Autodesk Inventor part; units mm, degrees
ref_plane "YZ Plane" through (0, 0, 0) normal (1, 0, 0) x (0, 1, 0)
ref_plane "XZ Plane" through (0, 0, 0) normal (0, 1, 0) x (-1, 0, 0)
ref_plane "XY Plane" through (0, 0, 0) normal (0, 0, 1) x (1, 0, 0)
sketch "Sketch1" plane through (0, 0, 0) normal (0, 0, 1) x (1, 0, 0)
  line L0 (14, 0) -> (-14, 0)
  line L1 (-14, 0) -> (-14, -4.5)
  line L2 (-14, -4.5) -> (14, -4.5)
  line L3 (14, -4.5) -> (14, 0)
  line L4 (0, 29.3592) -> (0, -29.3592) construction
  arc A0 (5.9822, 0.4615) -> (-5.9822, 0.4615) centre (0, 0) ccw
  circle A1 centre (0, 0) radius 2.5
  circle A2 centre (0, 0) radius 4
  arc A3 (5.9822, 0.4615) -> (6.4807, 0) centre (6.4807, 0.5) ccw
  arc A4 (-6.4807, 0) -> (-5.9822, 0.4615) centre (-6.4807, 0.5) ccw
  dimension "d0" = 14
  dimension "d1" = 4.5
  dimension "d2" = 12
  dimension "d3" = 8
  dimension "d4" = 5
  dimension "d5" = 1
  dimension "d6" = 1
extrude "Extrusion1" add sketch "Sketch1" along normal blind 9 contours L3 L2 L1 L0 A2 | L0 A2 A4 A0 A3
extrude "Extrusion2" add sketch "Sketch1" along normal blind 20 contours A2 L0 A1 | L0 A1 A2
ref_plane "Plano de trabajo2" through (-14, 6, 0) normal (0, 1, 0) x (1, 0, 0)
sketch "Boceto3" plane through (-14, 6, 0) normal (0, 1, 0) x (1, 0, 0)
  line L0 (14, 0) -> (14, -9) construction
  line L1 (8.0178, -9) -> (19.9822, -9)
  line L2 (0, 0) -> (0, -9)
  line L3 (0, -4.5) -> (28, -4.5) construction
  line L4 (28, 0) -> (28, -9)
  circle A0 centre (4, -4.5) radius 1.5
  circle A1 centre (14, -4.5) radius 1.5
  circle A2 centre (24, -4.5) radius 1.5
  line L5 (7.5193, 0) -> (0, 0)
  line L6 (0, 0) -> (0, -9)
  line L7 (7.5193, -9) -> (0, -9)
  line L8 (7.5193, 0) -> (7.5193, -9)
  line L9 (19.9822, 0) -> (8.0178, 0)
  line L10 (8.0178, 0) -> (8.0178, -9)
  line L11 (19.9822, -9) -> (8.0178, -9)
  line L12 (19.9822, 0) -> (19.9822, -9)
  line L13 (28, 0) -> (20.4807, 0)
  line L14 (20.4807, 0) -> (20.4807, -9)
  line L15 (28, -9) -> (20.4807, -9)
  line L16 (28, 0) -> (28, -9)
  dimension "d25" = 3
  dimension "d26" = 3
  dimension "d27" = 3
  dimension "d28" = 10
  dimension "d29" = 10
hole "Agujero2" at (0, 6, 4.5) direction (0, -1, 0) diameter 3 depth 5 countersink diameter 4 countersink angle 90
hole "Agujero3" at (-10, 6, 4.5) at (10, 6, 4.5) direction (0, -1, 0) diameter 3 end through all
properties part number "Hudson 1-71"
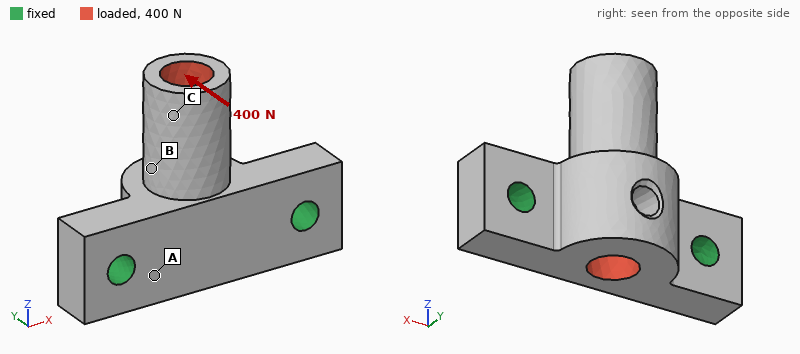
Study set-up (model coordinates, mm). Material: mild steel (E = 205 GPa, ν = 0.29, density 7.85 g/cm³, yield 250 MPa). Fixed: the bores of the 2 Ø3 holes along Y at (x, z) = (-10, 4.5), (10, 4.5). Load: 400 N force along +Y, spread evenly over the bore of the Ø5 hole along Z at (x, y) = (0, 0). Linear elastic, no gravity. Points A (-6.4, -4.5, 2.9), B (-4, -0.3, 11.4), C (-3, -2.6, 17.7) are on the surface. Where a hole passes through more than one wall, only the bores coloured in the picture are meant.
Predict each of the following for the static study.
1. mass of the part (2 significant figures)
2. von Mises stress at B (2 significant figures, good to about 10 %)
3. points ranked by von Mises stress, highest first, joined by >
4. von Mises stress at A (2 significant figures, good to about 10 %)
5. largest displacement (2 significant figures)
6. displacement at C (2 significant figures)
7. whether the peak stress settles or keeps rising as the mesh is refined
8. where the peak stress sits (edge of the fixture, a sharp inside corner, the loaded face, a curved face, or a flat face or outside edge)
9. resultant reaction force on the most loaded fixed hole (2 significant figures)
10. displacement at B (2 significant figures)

13 g
14 MPa
A > B > C
23 MPa
9.7 µm
7.9 µm
keeps rising
edge of the fixture
210 N
3.9 µm
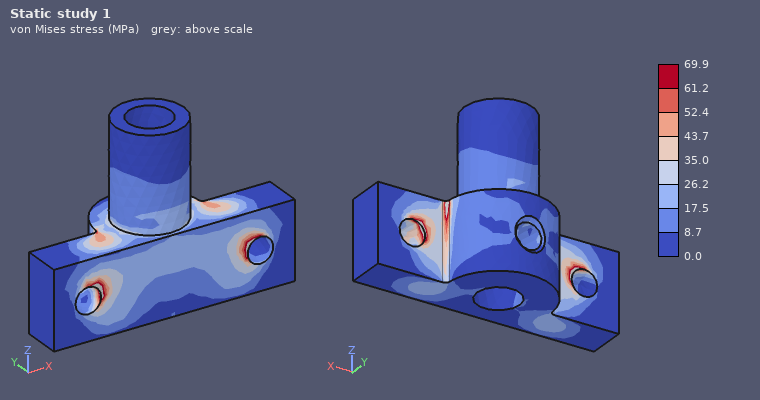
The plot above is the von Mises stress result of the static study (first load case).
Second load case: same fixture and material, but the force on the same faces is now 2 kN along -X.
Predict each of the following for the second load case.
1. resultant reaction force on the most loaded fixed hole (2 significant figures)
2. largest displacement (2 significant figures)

1.2 kN
19 µm
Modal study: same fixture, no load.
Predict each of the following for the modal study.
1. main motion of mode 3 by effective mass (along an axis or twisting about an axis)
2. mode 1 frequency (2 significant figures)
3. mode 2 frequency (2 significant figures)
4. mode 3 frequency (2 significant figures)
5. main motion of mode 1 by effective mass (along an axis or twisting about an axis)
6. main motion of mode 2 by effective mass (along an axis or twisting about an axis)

along Z
16 kHz
28 kHz
37 kHz
along Y
along X
